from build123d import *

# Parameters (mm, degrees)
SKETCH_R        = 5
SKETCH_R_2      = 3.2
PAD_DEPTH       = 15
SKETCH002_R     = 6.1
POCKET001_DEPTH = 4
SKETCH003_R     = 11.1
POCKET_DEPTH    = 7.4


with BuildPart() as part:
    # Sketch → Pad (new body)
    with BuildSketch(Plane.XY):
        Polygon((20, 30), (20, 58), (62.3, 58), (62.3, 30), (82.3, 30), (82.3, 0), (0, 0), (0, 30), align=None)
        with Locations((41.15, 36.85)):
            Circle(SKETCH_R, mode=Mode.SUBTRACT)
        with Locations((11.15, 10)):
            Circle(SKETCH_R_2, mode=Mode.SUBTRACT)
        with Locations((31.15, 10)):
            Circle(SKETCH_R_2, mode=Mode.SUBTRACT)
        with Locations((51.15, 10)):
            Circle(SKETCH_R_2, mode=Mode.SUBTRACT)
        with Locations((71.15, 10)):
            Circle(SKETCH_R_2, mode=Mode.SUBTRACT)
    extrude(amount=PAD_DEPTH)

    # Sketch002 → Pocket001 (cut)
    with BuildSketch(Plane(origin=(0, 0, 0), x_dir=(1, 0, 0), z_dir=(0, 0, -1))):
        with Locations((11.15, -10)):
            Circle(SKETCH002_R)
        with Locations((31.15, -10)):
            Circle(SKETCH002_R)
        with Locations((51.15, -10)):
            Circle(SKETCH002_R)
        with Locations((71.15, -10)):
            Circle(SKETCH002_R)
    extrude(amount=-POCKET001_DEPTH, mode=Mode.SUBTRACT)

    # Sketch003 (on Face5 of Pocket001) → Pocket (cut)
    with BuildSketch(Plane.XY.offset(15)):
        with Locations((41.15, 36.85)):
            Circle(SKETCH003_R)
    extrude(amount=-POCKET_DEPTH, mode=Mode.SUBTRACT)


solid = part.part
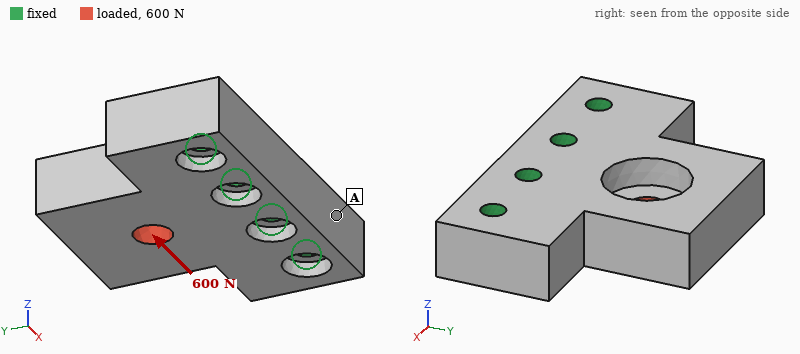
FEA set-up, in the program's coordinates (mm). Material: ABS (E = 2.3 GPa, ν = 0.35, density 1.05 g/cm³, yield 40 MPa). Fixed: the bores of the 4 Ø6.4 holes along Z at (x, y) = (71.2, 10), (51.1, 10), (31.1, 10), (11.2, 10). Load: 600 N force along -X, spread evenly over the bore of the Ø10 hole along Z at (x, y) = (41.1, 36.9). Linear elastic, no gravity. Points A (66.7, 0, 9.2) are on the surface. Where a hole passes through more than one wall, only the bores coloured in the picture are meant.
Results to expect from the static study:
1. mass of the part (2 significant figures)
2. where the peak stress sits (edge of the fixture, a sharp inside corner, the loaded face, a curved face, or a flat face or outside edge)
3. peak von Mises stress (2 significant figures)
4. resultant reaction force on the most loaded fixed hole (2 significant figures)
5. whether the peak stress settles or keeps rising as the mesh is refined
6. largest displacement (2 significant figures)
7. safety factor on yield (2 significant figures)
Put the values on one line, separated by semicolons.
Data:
50 g; the loaded face; 5.8 MPa; 270 N; settles; 55 µm; 6.9
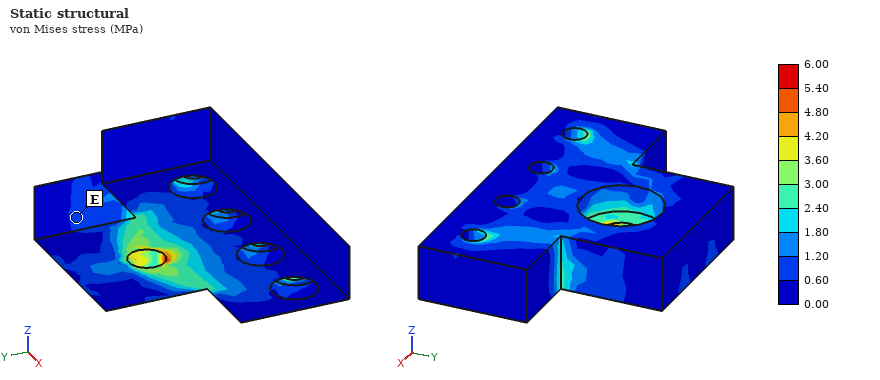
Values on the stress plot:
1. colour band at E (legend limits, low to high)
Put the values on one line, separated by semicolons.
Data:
0.60 to 1.20 MPa
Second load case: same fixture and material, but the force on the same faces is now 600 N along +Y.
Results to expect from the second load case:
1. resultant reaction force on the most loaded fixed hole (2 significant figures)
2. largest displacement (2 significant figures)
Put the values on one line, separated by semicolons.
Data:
220 N; 93 µm
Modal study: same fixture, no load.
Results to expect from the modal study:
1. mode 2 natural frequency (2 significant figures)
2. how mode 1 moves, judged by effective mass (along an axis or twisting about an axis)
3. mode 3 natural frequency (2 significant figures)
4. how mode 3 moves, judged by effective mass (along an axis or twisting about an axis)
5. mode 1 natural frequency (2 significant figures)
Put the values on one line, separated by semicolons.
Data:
3000 Hz; along Z; 3800 Hz; along X; 1400 Hz
